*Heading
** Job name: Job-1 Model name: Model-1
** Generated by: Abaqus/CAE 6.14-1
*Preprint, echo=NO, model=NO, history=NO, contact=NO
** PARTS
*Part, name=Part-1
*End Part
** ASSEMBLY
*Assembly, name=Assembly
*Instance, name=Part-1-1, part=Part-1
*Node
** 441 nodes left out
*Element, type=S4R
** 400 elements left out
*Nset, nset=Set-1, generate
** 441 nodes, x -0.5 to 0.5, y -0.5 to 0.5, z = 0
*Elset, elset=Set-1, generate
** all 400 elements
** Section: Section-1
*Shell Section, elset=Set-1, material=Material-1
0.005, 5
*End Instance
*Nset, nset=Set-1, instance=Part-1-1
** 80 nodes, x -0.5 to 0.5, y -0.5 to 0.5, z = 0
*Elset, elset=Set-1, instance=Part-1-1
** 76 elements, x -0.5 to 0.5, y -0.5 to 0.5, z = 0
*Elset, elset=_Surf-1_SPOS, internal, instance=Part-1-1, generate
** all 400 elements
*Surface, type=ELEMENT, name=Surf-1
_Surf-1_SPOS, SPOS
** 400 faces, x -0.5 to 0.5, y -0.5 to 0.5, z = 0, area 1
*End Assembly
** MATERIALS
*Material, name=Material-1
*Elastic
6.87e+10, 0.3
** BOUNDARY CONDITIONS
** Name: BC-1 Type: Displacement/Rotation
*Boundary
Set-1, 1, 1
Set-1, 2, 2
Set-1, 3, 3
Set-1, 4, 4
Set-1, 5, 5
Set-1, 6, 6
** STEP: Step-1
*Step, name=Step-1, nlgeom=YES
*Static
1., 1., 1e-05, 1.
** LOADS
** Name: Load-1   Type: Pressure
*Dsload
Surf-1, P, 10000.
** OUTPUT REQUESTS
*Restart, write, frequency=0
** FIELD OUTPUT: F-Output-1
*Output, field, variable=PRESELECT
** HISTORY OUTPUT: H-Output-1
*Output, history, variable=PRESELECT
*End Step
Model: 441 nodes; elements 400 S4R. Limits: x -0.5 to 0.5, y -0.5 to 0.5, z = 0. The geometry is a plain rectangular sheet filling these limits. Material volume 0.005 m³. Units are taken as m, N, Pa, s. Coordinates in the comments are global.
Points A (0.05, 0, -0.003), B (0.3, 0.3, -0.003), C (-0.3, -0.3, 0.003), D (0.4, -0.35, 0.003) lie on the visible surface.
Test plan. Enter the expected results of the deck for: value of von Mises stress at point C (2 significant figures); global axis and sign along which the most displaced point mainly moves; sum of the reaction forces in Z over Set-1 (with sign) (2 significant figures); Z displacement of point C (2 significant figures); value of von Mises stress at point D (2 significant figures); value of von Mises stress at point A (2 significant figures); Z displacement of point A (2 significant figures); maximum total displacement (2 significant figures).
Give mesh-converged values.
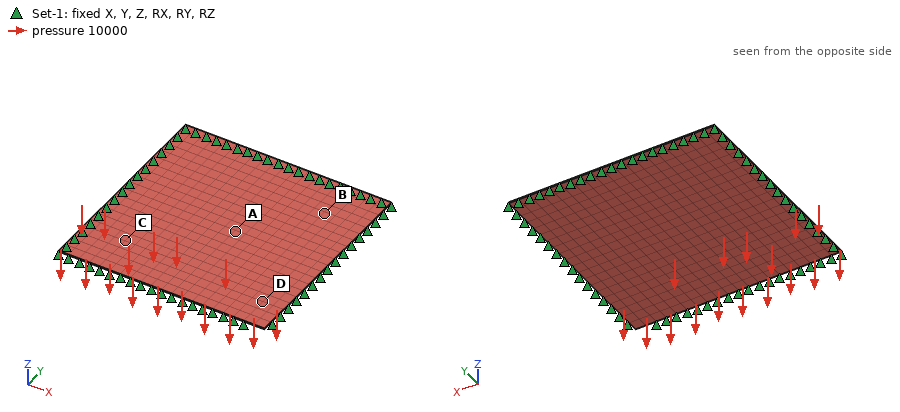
1.9e+07 Pa
-Z
10000 N
-0.0020 m
2.0e+07 Pa
3.1e+07 Pa
-0.0072 m
0.0073 m
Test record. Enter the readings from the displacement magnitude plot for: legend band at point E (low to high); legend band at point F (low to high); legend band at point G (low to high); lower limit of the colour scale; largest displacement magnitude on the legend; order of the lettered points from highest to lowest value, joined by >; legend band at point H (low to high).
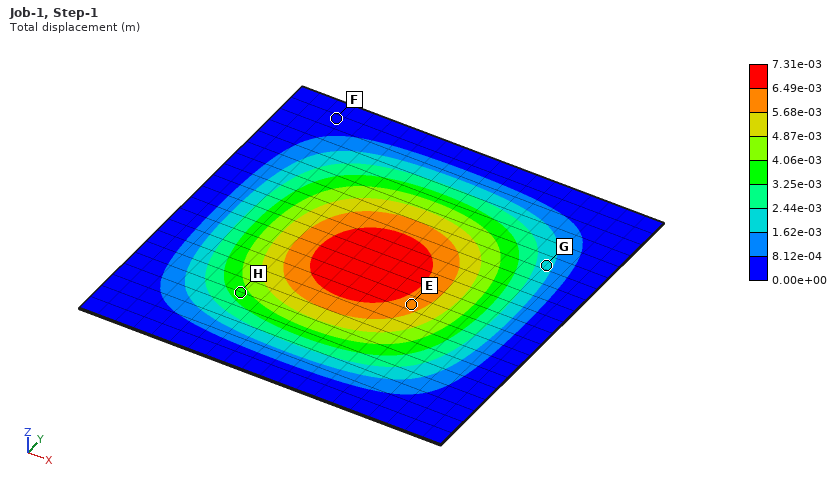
5.68e-03 to 6.49e-03 m
0.00e+00 to 8.12e-04 m
1.62e-03 to 2.44e-03 m
0.00e+00 m
7.31e-03 m
E > H > G > F
3.25e-03 to 4.06e-03 m
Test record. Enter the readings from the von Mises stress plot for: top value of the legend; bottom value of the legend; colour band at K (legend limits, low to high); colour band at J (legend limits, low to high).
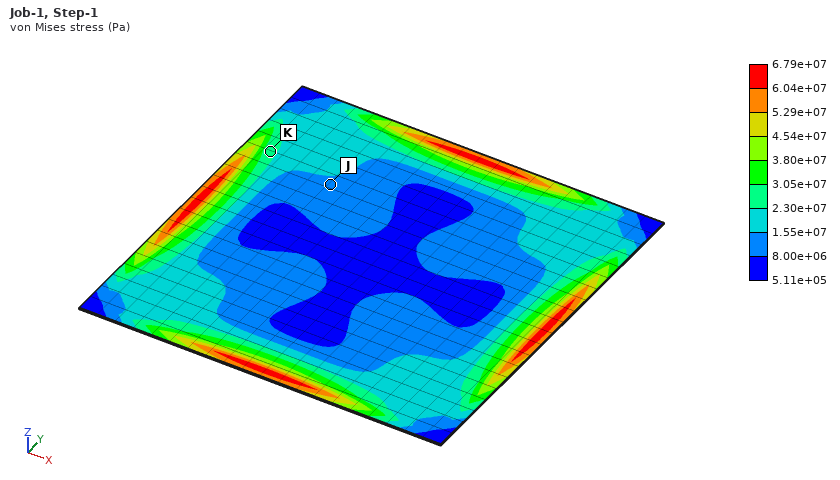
6.79e+07 Pa
5.11e+05 Pa
2.30e+07 to 3.05e+07 Pa
8.00e+06 to 1.55e+07 Pa
